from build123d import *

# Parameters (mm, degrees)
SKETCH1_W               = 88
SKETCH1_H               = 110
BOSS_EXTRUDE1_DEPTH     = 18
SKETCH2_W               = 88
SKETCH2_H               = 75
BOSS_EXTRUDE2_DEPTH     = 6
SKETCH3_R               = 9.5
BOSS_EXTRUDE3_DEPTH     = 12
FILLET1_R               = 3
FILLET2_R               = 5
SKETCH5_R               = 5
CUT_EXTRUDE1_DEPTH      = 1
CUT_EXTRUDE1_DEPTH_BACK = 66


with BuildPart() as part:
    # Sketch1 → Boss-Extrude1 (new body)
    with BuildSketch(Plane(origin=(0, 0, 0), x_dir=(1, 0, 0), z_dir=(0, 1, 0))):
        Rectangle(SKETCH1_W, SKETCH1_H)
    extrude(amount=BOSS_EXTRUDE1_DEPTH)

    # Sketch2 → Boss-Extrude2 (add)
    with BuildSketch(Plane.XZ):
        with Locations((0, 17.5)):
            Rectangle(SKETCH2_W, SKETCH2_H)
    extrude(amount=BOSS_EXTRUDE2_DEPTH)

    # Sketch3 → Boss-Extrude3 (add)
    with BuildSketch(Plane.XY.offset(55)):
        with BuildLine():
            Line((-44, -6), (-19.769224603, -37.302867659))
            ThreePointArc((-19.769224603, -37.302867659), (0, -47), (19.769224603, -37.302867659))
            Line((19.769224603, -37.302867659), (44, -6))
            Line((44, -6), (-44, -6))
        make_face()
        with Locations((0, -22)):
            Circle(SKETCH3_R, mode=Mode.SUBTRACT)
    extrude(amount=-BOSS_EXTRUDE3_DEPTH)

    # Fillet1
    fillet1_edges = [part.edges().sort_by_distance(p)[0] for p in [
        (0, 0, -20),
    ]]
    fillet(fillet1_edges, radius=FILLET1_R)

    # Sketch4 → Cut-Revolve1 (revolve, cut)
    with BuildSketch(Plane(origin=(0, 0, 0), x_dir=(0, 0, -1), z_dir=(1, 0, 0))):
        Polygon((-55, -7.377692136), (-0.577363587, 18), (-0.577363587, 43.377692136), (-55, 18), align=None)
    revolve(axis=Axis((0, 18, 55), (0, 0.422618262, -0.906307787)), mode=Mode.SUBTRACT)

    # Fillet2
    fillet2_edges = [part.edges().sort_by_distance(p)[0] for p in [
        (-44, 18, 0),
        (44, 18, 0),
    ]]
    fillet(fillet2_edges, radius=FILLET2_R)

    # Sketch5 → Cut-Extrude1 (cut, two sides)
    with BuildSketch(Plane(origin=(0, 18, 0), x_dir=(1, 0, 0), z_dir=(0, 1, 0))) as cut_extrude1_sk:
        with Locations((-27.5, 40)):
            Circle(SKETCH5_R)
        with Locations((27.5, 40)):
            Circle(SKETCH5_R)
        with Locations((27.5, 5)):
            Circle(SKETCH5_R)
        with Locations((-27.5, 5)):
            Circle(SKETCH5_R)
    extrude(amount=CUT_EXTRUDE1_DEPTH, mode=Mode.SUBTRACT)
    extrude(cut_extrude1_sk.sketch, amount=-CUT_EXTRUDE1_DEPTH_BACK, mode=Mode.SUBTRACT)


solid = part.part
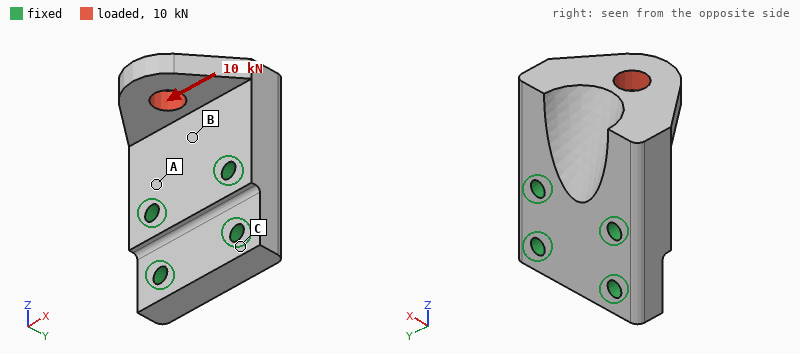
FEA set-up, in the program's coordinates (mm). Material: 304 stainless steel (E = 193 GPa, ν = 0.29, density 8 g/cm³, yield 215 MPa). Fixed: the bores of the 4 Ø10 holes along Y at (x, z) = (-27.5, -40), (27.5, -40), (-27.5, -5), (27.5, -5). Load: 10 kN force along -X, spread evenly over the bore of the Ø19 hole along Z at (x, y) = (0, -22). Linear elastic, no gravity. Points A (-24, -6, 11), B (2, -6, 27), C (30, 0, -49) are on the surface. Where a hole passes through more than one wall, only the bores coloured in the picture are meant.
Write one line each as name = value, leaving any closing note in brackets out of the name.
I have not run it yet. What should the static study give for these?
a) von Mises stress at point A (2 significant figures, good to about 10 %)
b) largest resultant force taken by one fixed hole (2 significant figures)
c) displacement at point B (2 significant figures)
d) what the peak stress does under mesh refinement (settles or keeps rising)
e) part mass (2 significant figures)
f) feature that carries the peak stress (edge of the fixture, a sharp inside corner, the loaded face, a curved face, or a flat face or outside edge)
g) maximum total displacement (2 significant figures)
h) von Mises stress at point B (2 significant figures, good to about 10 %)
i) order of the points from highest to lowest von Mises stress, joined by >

von Mises stress at point A = 28 MPa
largest resultant force taken by one fixed hole = 10 kN
displacement at point B = 6.0 µm
what the peak stress does under mesh refinement = keeps rising
part mass = 1.7 kg
feature that carries the peak stress = edge of the fixture
maximum total displacement = 34 µm
von Mises stress at point B = 40 MPa
order of the points from highest to lowest von Mises stress, joined by > = B > A > C
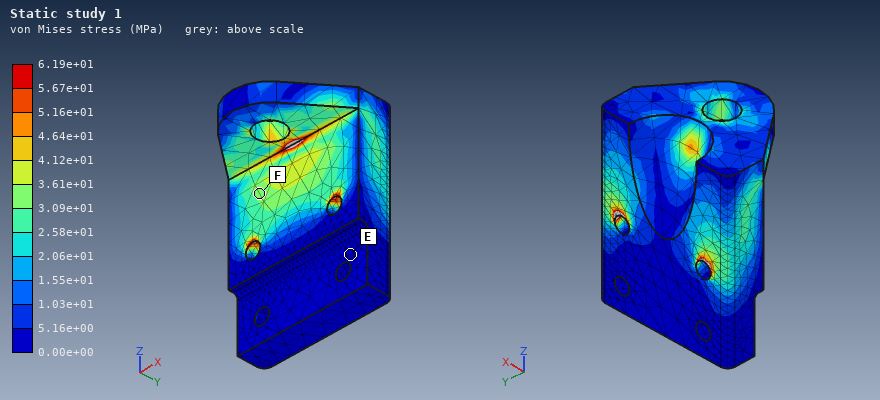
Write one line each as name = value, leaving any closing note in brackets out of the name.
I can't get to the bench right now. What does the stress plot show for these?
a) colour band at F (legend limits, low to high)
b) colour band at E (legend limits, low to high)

colour band at F = 3.09e+01 to 3.61e+01 MPa
colour band at E = 0.00e+00 to 5.16e+00 MPa
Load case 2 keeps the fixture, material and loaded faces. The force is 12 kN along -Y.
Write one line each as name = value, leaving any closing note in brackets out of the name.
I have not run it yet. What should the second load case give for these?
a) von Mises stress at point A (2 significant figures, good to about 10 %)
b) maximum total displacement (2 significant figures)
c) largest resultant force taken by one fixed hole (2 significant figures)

von Mises stress at point A = 67 MPa
maximum total displacement = 88 µm
largest resultant force taken by one fixed hole = 7.9 kN
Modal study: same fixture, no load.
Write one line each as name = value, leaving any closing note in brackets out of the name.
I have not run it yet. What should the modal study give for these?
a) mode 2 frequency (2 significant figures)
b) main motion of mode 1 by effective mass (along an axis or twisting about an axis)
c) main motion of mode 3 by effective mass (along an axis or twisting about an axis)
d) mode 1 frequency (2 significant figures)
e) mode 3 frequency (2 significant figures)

mode 2 frequency = 5000 Hz
main motion of mode 1 by effective mass = along Y
main motion of mode 3 by effective mass = along Y
mode 1 frequency = 3300 Hz
mode 3 frequency = 5700 Hz
